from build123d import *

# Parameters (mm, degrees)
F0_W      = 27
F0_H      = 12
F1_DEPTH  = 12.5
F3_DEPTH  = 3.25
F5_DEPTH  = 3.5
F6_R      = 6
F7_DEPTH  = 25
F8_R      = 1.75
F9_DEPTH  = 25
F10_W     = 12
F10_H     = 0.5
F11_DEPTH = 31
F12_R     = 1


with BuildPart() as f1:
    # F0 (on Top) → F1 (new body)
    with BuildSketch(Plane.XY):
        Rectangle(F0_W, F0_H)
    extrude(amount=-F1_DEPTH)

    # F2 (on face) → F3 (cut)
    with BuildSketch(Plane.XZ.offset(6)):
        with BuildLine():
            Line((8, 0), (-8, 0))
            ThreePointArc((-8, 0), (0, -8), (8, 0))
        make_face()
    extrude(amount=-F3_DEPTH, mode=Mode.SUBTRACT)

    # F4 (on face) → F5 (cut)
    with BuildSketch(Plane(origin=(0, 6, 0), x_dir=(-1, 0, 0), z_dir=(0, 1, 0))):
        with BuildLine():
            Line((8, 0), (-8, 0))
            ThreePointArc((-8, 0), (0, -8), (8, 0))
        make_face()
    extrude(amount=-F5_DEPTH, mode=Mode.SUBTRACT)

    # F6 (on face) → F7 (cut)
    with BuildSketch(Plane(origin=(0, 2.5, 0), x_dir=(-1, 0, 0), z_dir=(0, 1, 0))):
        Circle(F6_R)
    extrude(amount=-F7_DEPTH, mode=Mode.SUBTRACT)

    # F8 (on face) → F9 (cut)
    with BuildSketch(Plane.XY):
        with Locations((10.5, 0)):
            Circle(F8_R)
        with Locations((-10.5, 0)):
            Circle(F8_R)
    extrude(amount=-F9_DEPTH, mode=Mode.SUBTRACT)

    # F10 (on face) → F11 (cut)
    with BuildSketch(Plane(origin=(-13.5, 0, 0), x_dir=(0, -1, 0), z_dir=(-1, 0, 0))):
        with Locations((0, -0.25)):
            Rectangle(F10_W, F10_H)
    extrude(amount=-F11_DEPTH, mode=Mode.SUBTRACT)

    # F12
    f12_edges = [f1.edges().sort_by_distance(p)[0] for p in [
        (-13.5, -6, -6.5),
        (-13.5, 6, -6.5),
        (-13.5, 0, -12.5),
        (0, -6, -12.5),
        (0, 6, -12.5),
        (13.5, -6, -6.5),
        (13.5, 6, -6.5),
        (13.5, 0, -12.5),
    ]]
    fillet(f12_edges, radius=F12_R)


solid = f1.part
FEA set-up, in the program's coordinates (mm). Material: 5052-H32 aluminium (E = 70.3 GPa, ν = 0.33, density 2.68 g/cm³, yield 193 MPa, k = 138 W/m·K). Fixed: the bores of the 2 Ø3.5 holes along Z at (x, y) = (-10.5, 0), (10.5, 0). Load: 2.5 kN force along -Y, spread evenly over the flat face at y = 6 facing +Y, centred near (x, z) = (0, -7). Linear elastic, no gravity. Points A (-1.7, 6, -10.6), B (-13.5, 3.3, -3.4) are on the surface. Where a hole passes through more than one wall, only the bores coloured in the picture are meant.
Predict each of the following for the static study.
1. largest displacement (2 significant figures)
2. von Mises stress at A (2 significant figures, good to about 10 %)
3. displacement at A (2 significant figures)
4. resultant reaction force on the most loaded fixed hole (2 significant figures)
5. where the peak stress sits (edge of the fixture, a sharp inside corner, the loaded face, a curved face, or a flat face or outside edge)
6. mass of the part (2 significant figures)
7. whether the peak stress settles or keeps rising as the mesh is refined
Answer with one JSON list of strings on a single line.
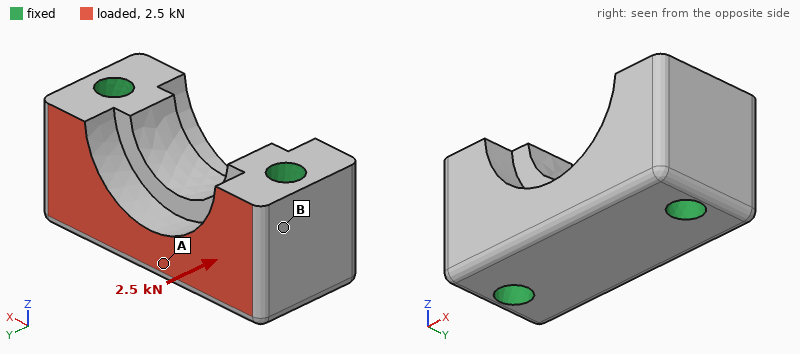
["3.2 µm", "12 MPa", "3.1 µm", "1.3 kN", "edge of the fixture", "7.3 g", "keeps rising"]
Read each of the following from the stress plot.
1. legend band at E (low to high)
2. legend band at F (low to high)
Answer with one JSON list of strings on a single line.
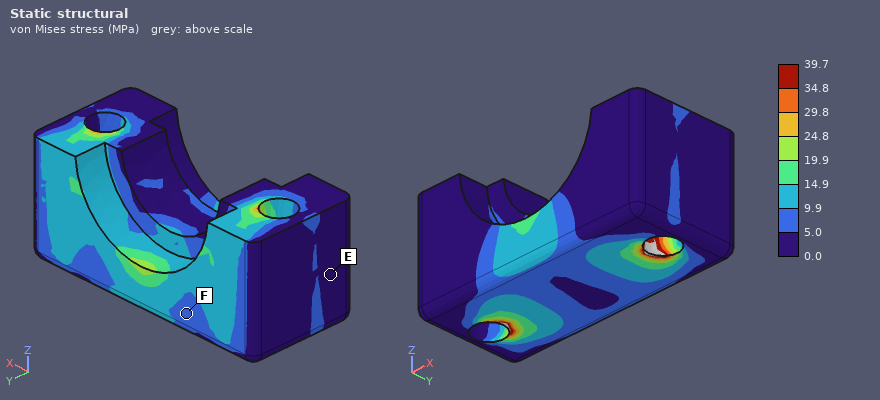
["0.0 to 5.0 MPa", "5.0 to 9.9 MPa"]
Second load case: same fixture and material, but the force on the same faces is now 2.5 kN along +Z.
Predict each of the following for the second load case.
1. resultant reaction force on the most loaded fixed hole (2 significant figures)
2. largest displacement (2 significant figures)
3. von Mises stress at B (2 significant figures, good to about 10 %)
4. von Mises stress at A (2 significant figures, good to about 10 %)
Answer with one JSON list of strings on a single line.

["1.3 kN", "8.4 µm", "17 MPa", "28 MPa"]
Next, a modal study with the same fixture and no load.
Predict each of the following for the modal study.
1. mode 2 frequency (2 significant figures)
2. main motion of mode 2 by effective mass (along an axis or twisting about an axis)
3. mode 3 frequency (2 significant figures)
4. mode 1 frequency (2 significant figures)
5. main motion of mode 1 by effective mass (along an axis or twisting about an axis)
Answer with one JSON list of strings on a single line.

["72 kHz", "along Z", "88 kHz", "60 kHz", "along Y"]
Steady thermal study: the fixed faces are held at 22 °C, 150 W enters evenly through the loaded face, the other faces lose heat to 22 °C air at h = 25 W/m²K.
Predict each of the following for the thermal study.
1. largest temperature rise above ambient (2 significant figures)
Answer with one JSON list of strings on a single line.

["39 K"]
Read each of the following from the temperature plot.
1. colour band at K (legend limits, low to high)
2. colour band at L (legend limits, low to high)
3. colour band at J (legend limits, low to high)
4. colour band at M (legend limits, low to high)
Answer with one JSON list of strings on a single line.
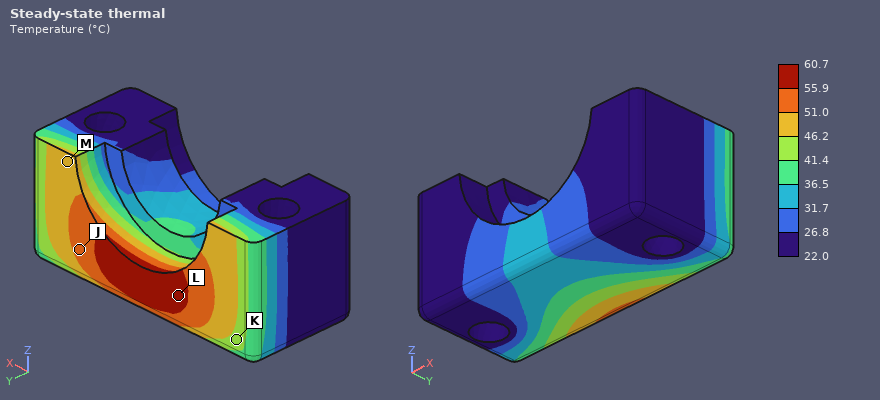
["41.4 to 46.2 °C", "55.9 to 60.7 °C", "51.0 to 55.9 °C", "46.2 to 51.0 °C"]
